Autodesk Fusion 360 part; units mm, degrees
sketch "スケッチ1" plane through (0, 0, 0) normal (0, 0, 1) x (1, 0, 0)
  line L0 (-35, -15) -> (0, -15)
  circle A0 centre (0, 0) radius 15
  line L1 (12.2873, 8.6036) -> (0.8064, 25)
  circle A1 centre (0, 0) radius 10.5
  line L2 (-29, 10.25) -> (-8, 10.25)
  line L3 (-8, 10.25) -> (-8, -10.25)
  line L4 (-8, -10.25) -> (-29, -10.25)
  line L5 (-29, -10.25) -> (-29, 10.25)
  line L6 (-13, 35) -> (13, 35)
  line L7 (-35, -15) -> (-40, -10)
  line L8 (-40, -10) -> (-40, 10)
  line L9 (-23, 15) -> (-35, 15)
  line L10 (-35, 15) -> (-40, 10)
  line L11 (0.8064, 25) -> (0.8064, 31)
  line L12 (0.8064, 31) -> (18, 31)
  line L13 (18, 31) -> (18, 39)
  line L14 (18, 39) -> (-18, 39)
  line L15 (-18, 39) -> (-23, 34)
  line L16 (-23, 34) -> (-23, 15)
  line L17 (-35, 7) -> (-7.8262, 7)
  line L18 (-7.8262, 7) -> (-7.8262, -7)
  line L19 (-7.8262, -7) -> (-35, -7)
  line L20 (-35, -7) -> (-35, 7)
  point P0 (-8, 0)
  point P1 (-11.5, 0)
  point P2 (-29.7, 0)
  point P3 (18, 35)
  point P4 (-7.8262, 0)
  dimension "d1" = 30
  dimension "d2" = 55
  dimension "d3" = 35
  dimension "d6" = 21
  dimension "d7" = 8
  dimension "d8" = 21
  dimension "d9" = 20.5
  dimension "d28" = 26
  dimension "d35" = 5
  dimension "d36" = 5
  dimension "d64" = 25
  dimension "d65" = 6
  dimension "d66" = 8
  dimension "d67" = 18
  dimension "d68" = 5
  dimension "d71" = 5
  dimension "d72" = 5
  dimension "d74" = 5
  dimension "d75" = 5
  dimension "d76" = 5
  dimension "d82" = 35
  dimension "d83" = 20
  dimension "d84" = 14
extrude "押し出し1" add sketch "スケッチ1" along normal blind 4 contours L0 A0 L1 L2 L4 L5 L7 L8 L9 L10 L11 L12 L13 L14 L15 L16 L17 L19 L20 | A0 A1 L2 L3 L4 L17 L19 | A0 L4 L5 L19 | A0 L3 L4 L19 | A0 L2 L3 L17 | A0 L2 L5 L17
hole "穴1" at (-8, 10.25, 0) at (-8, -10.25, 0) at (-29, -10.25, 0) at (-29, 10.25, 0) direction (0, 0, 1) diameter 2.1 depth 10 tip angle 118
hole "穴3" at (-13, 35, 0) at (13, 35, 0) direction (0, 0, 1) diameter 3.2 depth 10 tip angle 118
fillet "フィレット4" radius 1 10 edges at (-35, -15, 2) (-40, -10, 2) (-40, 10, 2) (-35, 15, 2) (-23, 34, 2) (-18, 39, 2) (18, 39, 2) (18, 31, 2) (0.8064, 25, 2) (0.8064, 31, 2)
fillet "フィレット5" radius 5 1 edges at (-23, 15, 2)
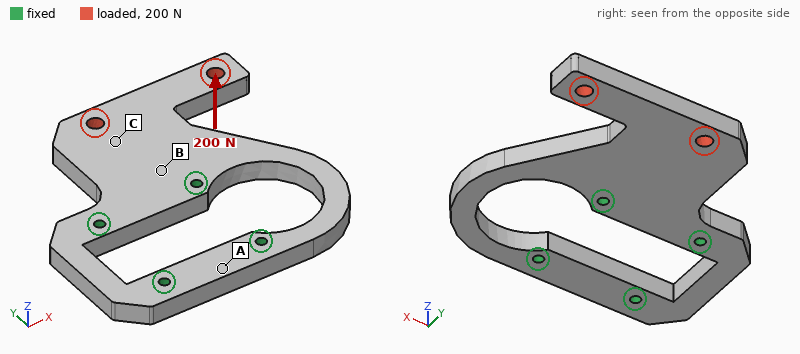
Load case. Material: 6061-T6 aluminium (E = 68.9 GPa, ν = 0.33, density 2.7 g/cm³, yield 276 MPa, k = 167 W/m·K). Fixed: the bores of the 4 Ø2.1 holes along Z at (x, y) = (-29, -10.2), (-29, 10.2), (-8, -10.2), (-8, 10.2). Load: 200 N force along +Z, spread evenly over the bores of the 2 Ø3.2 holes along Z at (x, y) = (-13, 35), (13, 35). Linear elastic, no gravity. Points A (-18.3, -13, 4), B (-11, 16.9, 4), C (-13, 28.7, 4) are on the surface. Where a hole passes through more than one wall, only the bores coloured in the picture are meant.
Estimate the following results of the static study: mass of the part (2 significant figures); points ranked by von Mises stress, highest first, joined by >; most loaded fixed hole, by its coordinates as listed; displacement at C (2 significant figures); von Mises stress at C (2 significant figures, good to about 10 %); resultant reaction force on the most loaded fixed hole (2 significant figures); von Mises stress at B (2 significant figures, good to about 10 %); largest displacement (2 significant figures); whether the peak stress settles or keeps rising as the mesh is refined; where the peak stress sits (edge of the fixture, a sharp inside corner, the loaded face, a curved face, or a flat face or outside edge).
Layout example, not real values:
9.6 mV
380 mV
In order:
17 g
B > C > A
(-8, 10.2)
0.085 mm
28 MPa
290 N
55 MPa
0.35 mm
keeps rising
edge of the fixture
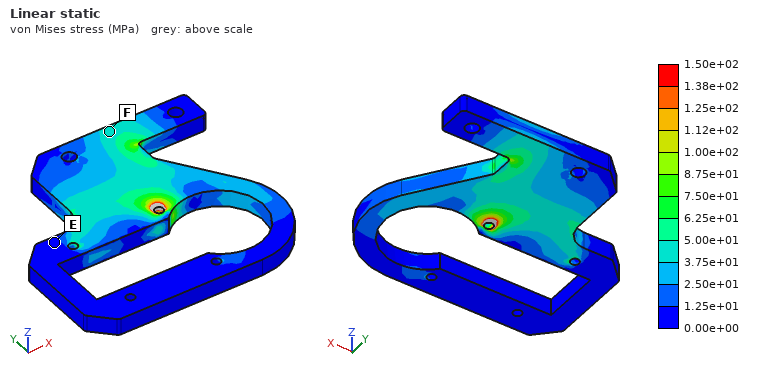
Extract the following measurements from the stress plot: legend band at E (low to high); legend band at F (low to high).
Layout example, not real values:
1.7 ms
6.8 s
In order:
0.00e+00 to 1.25e+01 MPa
3.75e+01 to 5.00e+01 MPa
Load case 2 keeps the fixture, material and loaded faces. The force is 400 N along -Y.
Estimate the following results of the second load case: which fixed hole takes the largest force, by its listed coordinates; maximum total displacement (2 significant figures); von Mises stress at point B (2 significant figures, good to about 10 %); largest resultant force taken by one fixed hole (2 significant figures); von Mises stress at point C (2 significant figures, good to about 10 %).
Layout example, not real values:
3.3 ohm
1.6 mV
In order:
(-8, 10.2)
57 µm
8.5 MPa
520 N
7.1 MPa
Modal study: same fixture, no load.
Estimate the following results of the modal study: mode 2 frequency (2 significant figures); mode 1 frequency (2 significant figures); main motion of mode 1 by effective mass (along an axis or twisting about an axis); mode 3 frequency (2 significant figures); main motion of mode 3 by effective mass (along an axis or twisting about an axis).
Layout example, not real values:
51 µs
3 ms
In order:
4800 Hz
2700 Hz
along Z
6200 Hz
along Z
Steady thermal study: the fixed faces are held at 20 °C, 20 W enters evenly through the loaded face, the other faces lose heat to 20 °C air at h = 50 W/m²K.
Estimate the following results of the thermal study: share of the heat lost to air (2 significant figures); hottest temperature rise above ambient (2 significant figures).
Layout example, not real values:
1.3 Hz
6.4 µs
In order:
14 %
59 K
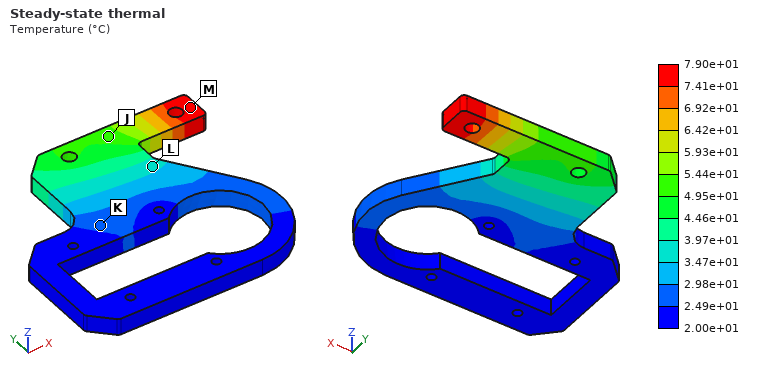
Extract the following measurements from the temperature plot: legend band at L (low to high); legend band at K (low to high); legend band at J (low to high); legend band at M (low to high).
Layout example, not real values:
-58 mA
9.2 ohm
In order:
3.47e+01 to 3.97e+01 °C
2.49e+01 to 2.98e+01 °C
4.95e+01 to 5.44e+01 °C
7.41e+01 to 7.90e+01 °C
